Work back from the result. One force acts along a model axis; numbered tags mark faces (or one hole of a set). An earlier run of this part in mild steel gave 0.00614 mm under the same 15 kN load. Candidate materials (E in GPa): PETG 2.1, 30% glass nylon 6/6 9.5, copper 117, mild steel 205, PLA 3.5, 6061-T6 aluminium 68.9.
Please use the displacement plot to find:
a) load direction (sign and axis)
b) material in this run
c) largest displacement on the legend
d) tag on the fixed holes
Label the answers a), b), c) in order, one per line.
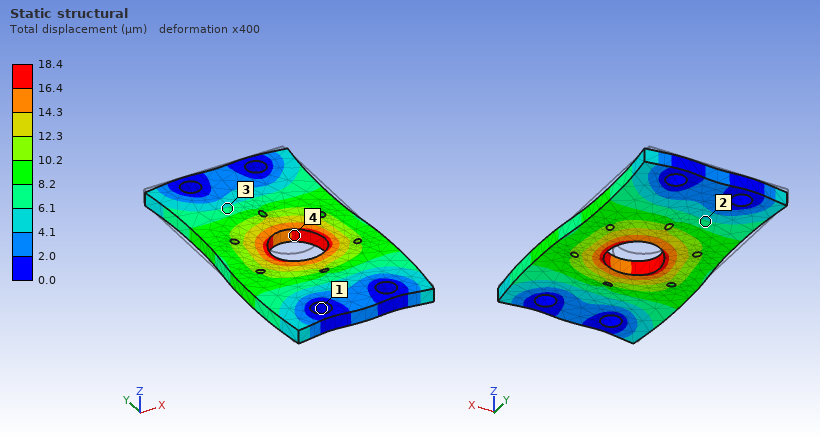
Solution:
a) -Y
b) 6061-T6 aluminium
c) 18.4 µm
d) 1
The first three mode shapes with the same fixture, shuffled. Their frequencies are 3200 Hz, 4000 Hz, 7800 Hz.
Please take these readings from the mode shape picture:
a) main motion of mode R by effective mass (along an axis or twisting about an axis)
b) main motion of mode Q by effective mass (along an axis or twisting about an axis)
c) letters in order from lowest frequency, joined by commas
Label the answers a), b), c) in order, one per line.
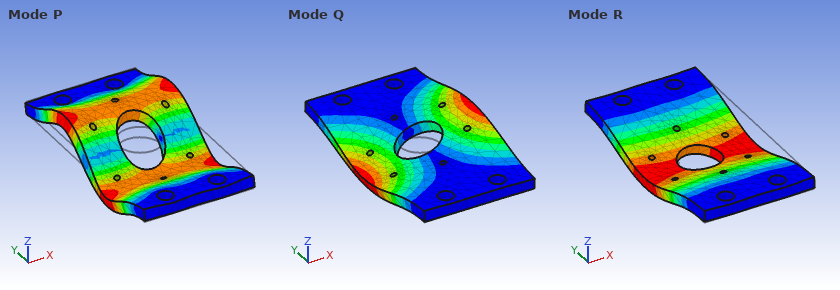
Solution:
a) along Z
b) twisting about Y
c) R, Q, P
